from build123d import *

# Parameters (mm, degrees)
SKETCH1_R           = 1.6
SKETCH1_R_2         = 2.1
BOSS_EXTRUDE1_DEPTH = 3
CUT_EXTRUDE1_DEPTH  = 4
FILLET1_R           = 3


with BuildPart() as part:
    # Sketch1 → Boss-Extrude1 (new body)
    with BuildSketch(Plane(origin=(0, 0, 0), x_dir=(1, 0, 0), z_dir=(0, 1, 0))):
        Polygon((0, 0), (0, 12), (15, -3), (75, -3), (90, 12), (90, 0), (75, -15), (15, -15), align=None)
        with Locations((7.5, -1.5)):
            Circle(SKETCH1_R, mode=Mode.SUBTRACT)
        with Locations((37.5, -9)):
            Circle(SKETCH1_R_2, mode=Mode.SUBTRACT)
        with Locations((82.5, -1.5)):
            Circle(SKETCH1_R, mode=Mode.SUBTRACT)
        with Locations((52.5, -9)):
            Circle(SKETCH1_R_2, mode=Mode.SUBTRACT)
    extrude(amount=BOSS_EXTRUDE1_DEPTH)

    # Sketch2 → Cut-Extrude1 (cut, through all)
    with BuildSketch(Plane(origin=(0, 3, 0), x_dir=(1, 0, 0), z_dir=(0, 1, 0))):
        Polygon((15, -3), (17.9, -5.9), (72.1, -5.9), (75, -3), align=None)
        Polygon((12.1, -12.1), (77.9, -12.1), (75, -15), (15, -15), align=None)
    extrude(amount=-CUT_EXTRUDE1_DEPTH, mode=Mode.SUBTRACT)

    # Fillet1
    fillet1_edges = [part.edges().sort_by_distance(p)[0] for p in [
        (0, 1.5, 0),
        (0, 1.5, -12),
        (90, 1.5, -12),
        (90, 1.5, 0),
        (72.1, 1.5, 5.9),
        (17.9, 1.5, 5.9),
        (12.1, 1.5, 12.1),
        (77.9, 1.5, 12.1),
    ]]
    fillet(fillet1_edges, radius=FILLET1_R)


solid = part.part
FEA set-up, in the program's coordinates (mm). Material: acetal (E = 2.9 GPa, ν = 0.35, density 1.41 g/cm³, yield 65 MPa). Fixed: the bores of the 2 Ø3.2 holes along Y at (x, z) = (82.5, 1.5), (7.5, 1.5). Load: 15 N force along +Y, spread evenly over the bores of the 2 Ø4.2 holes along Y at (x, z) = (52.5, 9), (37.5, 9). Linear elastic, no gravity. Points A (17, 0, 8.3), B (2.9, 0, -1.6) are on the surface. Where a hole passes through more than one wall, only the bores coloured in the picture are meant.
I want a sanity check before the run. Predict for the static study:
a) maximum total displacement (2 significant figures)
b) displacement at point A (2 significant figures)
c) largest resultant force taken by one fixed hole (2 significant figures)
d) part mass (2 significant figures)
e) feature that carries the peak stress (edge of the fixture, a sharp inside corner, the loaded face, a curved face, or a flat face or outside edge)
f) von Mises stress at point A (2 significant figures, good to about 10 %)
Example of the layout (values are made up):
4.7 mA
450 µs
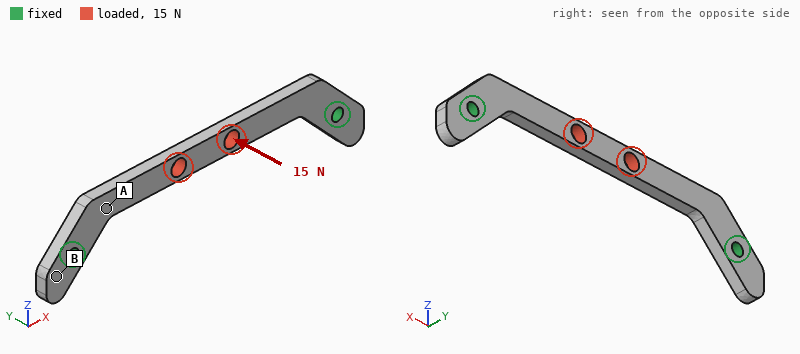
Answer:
0.87 mm
0.15 mm
7.5 N
2.8 g
the loaded face
8.4 MPa
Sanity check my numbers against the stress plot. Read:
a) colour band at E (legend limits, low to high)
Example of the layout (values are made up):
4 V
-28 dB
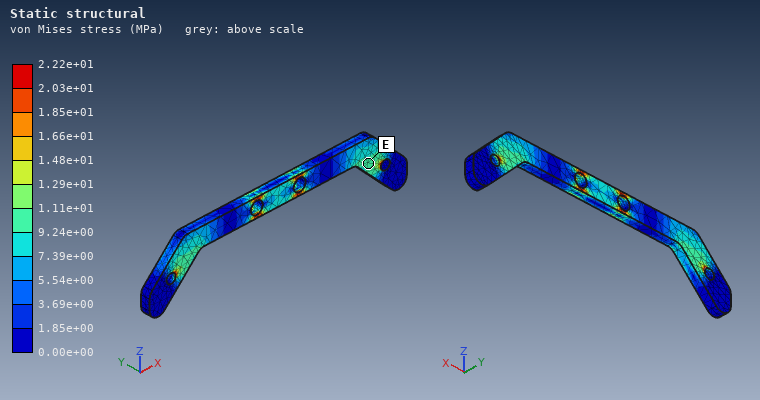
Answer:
9.24e+00 to 1.11e+01 MPa
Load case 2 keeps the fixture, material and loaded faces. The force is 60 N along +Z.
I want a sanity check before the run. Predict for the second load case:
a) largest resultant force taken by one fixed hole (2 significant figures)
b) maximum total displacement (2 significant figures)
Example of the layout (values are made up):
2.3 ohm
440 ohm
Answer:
56 N
0.56 mm
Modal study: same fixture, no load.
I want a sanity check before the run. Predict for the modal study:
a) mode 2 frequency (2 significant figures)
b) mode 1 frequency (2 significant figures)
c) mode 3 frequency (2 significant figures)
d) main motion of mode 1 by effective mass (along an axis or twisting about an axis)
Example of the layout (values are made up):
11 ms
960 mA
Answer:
2000 Hz
780 Hz
2000 Hz
along Y
